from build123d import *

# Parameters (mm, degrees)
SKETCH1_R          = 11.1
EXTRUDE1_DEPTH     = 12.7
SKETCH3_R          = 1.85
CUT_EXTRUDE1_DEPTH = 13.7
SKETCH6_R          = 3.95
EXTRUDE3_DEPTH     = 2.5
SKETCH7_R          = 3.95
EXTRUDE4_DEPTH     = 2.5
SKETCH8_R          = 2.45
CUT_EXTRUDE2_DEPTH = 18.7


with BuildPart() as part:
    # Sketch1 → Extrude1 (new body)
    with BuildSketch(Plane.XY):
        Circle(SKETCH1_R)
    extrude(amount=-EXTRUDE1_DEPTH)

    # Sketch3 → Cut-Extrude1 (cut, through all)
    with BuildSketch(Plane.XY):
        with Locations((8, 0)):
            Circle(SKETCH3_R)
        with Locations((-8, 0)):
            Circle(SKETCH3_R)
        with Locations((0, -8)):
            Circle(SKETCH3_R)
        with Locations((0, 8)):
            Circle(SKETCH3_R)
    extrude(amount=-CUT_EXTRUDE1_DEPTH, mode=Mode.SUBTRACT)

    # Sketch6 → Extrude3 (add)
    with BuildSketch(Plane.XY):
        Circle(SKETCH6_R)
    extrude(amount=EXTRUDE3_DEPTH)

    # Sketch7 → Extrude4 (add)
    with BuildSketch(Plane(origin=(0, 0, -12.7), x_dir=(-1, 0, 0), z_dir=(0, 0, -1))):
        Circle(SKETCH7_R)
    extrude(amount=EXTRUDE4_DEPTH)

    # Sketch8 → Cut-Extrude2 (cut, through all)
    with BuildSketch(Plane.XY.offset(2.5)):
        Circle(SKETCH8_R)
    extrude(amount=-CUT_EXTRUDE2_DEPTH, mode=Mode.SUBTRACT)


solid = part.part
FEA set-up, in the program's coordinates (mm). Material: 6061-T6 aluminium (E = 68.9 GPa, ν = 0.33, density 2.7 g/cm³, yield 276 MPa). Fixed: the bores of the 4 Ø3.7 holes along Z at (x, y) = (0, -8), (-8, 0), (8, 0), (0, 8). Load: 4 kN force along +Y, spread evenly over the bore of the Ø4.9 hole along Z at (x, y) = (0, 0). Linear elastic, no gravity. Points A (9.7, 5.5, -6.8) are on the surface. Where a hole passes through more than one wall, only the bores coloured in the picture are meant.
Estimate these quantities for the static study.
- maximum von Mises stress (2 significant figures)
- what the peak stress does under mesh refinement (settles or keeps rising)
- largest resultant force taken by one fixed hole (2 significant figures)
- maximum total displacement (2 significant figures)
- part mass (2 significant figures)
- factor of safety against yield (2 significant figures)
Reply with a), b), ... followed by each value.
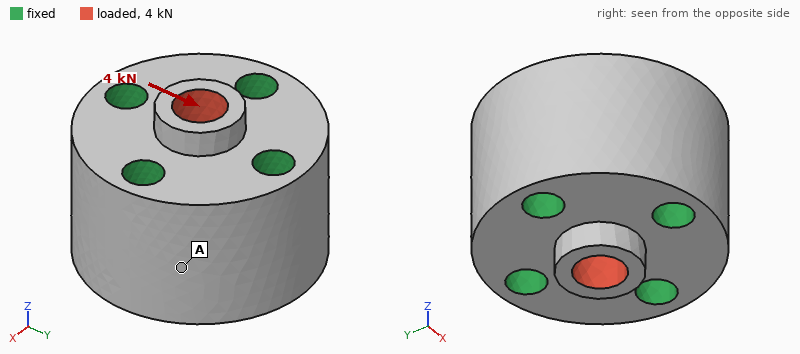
a) 56 MPa
b) settles
c) 1.4 kN
d) 4.7 µm
e) 12 g
f) 4.9
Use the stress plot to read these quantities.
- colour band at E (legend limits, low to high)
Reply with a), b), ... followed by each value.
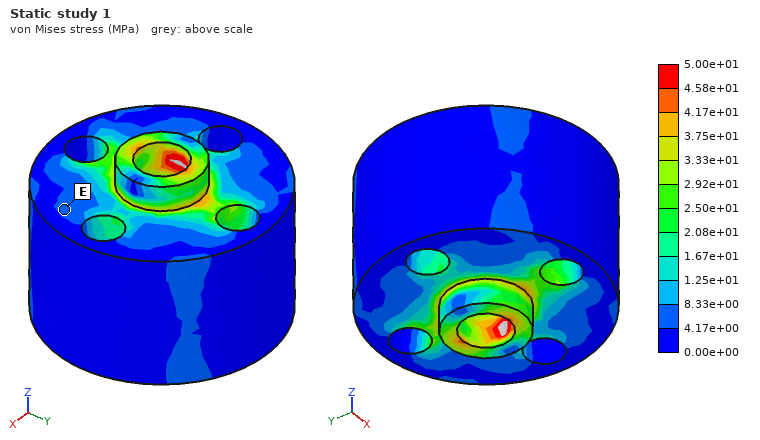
a) 4.17e+00 to 8.33e+00 MPa
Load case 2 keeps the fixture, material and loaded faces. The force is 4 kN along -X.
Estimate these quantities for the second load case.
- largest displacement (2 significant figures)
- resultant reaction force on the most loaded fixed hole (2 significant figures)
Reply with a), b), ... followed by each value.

a) 4.8 µm
b) 1.4 kN
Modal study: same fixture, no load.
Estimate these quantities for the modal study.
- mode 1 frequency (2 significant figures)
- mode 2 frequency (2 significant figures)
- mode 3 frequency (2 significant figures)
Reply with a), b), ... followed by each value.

a) 130 kHz
b) 130 kHz
c) 130 kHz
